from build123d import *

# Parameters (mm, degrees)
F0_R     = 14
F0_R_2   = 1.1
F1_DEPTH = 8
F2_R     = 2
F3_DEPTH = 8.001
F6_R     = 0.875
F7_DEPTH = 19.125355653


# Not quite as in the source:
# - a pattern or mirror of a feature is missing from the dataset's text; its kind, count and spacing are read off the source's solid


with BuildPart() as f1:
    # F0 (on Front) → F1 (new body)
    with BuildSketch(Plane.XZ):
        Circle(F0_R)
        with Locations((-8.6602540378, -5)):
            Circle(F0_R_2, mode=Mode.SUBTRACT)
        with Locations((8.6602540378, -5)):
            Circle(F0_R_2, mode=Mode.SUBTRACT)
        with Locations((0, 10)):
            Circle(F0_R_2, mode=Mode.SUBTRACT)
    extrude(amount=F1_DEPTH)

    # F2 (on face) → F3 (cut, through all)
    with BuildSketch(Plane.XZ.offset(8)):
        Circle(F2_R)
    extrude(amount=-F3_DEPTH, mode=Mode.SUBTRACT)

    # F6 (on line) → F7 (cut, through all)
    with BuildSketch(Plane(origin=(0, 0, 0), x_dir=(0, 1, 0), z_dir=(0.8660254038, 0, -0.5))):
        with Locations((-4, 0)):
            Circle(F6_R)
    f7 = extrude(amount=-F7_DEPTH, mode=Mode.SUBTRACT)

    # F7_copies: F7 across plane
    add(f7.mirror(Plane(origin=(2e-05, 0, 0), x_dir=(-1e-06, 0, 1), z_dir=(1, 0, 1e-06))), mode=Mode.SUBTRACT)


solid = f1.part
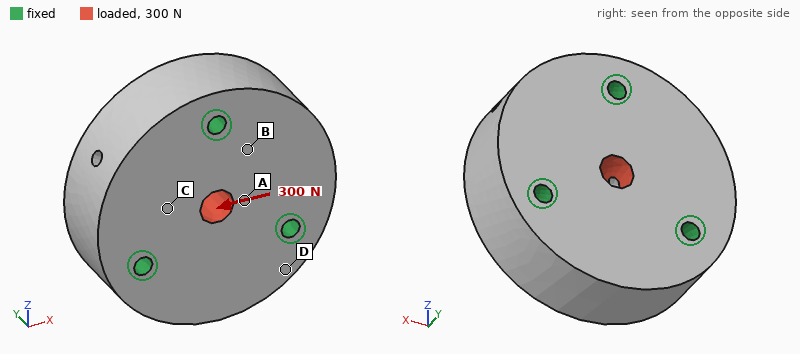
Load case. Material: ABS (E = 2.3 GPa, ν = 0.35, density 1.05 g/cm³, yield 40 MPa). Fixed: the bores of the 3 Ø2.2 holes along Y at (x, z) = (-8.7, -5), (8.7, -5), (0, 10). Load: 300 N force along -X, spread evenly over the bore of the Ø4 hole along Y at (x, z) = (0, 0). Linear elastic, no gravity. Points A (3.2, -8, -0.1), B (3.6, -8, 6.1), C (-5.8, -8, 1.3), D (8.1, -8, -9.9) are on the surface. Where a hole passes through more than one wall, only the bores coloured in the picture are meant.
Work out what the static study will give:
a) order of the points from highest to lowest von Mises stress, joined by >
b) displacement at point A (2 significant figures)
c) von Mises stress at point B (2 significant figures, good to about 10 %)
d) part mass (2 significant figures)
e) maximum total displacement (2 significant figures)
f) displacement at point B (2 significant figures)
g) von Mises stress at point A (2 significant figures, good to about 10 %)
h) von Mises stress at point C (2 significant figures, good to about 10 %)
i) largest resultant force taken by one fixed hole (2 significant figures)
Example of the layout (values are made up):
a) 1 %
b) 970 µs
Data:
a) A > C > B > D
b) 8.9 µm
c) 1.1 MPa
d) 4.9 g
e) 12 µm
f) 5.0 µm
g) 3.0 MPa
h) 1.5 MPa
i) 110 N
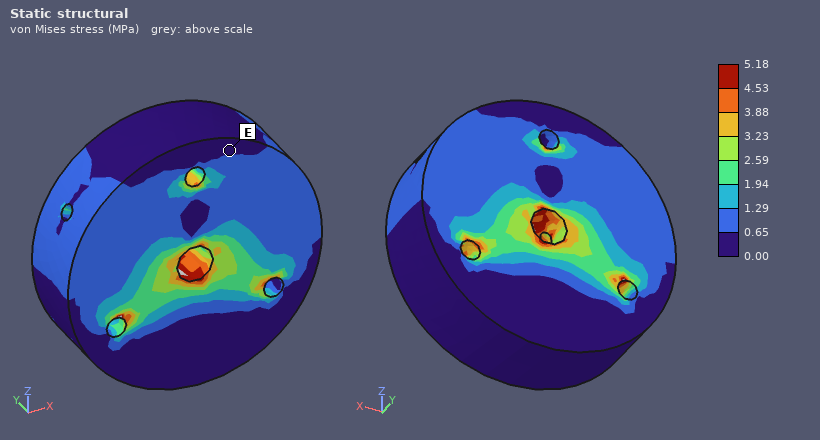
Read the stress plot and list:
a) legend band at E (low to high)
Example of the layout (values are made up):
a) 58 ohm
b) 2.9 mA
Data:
a) 0.00 to 0.65 MPa
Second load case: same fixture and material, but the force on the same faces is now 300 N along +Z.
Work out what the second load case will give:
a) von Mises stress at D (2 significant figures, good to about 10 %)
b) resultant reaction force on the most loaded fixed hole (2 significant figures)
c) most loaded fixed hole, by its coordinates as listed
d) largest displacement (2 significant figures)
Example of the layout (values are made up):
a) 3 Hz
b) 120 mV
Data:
a) 0.67 MPa
b) 110 N
c) (0, 10)
d) 12 µm
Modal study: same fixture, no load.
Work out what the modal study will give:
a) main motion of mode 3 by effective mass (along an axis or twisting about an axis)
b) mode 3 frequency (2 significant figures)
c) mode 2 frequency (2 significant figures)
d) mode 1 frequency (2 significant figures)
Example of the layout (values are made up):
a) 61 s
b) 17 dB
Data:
a) along Y
b) 15 kHz
c) 14 kHz
d) 14 kHz
